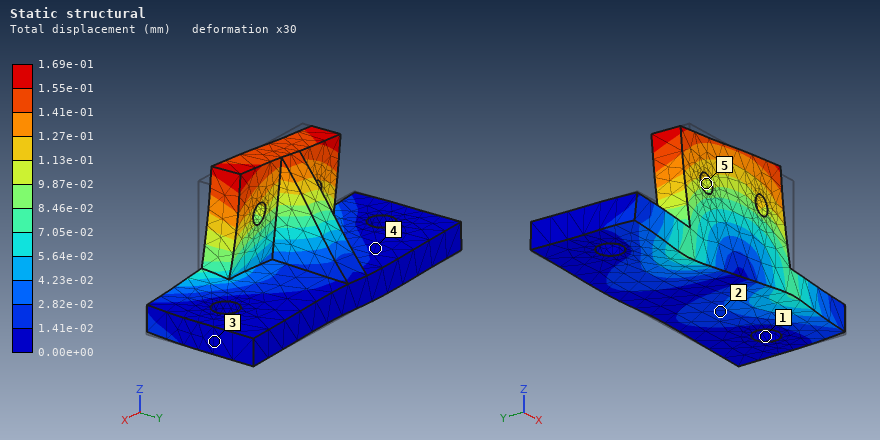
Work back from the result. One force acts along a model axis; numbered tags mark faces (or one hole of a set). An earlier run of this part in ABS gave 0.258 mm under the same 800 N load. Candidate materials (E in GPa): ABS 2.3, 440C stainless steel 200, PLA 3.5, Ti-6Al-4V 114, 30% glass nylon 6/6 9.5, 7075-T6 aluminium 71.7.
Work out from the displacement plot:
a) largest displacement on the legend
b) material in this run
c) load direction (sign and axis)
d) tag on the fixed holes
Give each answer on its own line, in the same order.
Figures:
1.69e-01 mm
PLA
-X
1
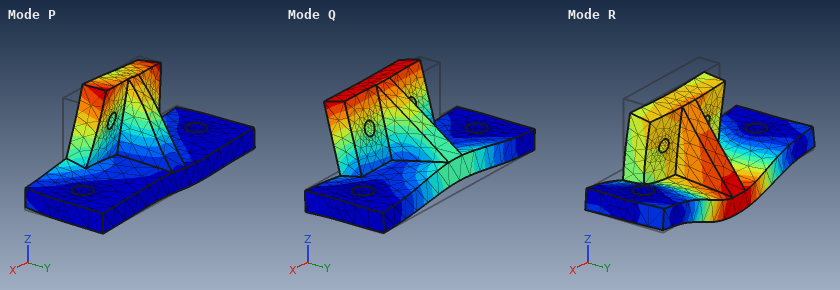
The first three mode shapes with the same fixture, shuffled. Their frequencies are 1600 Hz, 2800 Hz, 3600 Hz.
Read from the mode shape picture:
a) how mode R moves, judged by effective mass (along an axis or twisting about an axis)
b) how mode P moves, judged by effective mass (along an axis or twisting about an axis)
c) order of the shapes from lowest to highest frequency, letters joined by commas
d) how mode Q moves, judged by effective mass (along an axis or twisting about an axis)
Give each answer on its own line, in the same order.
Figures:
along Z
along X
Q, R, P
along Y
